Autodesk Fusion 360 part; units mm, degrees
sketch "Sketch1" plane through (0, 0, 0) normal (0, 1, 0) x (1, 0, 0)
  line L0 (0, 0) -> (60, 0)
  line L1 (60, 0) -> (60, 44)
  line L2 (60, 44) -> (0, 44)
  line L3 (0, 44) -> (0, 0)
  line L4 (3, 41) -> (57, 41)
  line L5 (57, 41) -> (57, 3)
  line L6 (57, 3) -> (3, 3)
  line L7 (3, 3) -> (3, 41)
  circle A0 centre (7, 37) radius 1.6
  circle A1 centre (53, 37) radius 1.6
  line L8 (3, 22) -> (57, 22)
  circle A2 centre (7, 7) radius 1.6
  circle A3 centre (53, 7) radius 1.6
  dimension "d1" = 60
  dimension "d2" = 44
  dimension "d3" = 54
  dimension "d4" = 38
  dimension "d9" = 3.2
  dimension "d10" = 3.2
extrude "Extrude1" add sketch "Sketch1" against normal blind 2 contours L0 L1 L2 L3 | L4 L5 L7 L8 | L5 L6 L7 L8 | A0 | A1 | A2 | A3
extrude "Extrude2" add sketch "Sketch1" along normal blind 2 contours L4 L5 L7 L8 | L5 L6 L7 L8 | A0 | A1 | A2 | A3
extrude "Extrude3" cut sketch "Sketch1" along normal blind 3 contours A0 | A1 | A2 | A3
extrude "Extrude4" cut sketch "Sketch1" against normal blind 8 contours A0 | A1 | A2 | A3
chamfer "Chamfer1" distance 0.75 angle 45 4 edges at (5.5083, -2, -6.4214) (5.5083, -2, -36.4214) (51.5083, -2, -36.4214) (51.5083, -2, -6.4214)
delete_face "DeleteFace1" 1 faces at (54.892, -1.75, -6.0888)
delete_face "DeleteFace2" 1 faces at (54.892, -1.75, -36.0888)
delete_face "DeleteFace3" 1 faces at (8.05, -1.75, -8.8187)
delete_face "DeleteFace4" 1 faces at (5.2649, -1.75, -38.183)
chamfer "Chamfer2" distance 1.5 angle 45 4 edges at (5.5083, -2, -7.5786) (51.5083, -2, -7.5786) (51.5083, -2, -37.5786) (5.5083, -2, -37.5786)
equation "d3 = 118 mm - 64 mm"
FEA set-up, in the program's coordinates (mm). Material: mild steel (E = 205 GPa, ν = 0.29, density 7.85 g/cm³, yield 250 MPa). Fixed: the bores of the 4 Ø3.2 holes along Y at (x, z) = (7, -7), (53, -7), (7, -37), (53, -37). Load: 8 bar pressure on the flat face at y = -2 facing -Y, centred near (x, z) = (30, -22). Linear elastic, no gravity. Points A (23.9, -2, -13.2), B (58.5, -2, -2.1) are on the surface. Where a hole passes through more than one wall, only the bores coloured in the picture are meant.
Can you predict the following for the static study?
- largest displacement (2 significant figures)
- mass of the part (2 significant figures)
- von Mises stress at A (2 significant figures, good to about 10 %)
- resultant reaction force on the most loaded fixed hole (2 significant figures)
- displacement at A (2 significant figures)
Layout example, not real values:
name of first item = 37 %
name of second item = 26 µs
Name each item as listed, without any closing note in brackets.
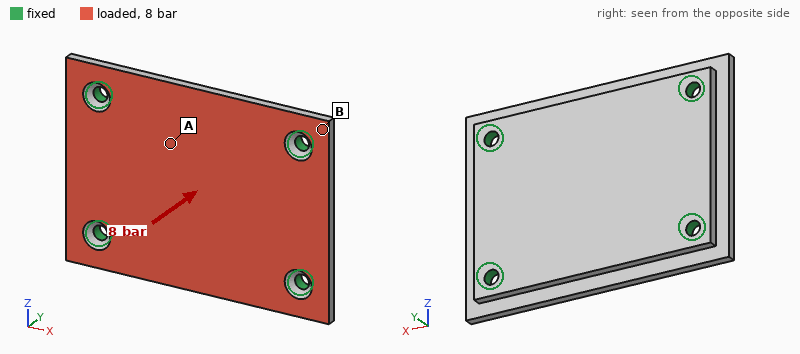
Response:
largest displacement = 17 µm
mass of the part = 72 g
von Mises stress at A = 30 MPa
resultant reaction force on the most loaded fixed hole = 550 N
displacement at A = 15 µm
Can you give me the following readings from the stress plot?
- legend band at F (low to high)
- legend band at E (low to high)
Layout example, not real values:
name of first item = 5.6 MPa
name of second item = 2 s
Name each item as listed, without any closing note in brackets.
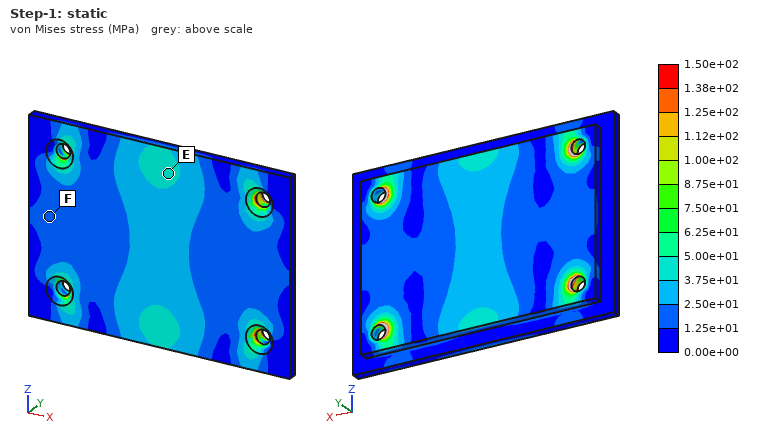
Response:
legend band at F = 1.25e+01 to 2.50e+01 MPa
legend band at E = 3.75e+01 to 5.00e+01 MPa
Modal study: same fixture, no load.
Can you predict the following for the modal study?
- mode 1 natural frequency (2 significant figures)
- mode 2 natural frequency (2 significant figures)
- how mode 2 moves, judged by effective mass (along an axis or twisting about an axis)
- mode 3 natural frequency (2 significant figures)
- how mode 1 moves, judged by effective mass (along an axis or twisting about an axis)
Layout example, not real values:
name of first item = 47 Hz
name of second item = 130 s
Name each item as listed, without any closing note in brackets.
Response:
mode 1 natural frequency = 7200 Hz
mode 2 natural frequency = 10 kHz
how mode 2 moves, judged by effective mass = twisting about X
mode 3 natural frequency = 16 kHz
how mode 1 moves, judged by effective mass = along Y
